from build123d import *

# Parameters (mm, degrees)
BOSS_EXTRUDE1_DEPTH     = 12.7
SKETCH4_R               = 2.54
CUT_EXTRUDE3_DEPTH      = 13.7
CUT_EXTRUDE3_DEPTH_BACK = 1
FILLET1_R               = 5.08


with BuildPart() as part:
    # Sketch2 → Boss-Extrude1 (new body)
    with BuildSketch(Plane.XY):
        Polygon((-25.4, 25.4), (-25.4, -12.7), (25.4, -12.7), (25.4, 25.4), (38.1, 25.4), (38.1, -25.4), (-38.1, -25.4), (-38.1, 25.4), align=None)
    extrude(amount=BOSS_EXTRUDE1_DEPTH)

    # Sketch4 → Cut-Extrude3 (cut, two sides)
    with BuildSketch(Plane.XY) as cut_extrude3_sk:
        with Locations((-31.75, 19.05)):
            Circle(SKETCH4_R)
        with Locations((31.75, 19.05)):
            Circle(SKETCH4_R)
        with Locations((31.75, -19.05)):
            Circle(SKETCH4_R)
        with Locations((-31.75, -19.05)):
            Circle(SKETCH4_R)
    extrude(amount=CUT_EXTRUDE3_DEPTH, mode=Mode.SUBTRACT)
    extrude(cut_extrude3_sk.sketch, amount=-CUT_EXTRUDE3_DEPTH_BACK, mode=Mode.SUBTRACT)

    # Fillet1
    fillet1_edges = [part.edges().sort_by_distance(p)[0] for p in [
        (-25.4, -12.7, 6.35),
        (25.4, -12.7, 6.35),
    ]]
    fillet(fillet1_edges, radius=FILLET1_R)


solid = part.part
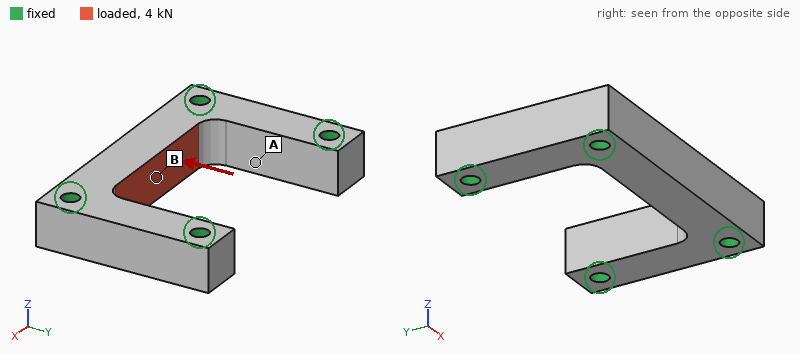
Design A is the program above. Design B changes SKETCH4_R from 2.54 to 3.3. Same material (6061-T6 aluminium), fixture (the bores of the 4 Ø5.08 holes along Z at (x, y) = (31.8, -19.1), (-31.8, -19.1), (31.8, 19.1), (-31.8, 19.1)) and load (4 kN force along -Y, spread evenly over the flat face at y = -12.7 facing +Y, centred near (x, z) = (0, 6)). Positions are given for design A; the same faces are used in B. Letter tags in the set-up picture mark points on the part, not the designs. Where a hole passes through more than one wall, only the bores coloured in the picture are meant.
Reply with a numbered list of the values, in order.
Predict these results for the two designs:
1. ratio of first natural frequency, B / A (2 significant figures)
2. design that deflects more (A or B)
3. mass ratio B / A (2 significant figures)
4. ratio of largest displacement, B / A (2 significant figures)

1. 1.1
2. A
3. 0.97
4. 0.90
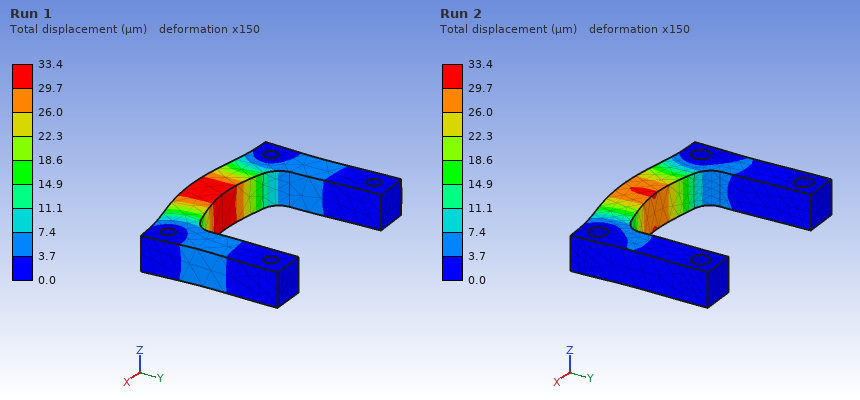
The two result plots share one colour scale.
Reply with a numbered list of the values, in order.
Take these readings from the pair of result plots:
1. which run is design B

1. Run 2
